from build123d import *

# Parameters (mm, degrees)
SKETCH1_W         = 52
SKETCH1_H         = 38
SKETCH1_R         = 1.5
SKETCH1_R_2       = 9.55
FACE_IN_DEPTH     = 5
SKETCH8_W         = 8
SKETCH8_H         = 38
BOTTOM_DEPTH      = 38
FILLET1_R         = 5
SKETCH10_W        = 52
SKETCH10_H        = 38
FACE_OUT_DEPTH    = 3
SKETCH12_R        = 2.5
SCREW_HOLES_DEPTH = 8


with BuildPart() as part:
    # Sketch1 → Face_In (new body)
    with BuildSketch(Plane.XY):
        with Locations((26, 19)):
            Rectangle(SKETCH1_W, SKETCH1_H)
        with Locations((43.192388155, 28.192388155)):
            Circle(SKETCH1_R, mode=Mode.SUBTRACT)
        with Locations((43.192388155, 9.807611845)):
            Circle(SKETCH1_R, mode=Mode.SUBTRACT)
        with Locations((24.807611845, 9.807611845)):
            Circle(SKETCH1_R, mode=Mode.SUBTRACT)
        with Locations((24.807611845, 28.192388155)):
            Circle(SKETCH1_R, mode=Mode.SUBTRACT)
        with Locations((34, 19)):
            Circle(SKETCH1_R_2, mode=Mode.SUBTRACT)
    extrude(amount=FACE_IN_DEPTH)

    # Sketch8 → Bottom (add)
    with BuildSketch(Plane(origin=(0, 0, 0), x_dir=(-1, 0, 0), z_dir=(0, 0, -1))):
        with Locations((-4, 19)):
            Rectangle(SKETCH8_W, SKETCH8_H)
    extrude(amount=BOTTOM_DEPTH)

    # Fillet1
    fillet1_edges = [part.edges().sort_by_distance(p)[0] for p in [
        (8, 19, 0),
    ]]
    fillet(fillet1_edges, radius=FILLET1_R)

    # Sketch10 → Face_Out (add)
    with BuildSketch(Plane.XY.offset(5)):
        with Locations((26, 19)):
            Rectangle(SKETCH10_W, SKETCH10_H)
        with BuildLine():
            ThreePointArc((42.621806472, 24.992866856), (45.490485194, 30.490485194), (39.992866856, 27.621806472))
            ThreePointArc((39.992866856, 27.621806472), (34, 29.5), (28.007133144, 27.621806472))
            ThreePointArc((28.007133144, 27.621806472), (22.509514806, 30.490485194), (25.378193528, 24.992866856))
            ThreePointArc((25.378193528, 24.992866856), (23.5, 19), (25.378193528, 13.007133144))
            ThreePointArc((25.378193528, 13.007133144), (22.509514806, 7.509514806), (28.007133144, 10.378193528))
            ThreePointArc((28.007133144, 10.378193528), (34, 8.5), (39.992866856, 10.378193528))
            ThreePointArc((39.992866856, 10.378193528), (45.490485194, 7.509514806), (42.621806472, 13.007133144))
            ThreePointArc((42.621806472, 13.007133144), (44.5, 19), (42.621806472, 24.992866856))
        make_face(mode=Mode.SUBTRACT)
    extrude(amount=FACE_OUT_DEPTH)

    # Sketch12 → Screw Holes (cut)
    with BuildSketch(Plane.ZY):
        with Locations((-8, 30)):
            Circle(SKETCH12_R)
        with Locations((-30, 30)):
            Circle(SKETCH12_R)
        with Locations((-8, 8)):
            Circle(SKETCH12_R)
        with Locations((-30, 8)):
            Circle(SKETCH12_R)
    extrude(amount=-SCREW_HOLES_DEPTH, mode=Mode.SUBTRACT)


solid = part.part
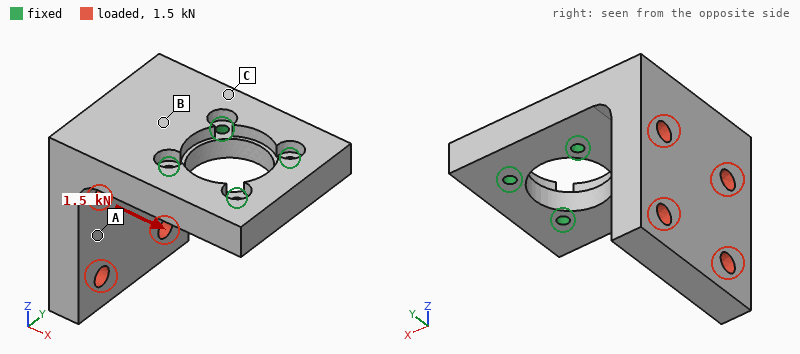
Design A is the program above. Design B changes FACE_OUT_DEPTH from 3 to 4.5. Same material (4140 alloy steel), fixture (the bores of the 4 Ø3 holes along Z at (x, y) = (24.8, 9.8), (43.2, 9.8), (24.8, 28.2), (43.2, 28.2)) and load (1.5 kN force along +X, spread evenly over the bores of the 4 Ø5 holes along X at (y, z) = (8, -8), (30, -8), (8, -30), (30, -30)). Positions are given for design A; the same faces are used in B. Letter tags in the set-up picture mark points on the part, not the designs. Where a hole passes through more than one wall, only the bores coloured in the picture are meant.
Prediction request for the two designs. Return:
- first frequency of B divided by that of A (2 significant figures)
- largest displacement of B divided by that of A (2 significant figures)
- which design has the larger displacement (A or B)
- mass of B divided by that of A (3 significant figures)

1.1
0.78
A
1.09
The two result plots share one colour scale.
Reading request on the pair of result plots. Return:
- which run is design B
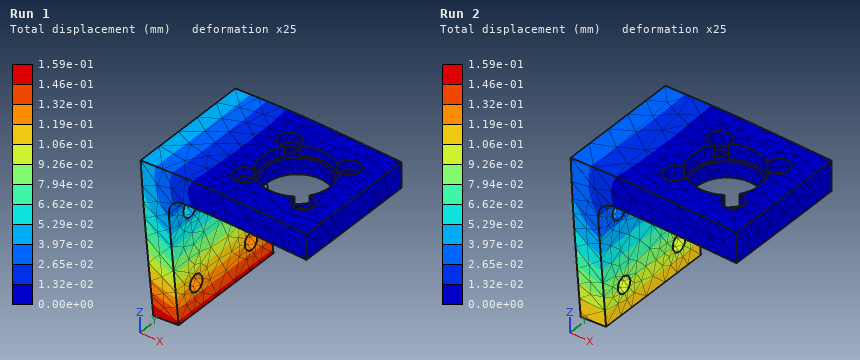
Run 2
